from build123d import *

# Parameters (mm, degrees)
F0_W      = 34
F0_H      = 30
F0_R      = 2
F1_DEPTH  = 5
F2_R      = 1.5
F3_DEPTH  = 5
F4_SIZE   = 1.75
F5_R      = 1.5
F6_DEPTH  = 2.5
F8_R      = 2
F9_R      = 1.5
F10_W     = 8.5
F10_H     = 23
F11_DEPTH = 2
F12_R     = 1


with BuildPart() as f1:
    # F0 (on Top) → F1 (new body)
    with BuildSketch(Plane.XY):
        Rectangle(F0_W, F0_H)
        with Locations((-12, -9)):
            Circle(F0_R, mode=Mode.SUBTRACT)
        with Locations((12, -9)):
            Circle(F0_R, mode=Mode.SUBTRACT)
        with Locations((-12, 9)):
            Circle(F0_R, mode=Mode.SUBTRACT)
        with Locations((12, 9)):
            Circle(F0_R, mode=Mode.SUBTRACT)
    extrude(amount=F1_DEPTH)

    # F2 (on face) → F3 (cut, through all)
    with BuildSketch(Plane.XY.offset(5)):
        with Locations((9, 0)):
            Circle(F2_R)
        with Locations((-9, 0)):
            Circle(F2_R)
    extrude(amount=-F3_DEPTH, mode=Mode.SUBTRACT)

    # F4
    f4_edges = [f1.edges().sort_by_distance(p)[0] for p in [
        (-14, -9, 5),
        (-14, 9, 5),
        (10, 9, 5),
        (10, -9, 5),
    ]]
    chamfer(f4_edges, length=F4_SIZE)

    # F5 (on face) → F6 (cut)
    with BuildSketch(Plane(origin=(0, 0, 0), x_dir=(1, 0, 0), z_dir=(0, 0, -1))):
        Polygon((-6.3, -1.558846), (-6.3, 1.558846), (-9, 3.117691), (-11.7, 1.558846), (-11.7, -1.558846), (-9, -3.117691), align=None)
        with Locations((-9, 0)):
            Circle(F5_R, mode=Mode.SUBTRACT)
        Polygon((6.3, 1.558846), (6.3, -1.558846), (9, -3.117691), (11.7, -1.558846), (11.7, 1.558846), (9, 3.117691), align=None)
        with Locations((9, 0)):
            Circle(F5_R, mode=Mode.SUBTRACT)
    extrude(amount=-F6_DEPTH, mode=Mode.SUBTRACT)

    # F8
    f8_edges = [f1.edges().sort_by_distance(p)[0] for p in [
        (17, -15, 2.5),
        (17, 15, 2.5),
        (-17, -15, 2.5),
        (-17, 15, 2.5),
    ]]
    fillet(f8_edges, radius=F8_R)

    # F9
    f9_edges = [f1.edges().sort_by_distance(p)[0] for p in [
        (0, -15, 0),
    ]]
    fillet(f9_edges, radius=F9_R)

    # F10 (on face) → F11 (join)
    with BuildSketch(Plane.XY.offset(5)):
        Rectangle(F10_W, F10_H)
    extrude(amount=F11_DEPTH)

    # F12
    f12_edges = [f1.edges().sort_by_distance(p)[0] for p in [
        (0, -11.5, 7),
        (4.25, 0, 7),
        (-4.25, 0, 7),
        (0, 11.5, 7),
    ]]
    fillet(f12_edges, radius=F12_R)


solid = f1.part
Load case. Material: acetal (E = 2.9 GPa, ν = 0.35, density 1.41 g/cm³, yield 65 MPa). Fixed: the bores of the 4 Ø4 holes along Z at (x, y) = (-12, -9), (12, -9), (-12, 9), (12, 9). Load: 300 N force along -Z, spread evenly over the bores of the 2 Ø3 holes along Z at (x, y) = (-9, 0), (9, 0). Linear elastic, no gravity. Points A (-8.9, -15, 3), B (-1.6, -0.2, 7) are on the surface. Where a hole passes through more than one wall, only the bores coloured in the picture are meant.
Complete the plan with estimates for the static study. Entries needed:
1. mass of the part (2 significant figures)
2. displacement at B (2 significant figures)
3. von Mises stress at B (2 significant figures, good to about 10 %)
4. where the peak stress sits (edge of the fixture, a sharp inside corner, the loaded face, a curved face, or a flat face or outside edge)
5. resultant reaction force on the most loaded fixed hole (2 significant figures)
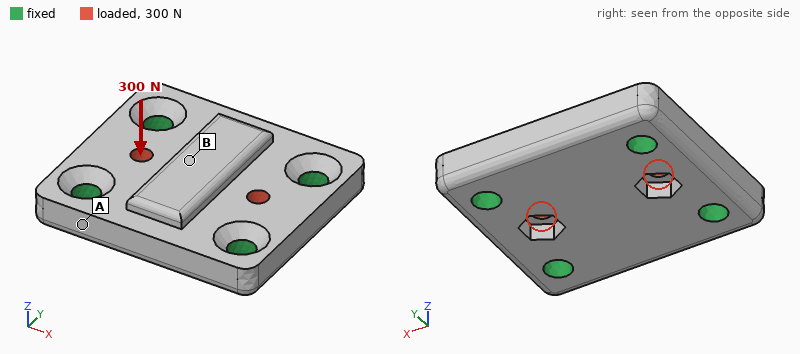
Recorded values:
6.9 g
23 µm
3.7 MPa
the loaded face
87 N
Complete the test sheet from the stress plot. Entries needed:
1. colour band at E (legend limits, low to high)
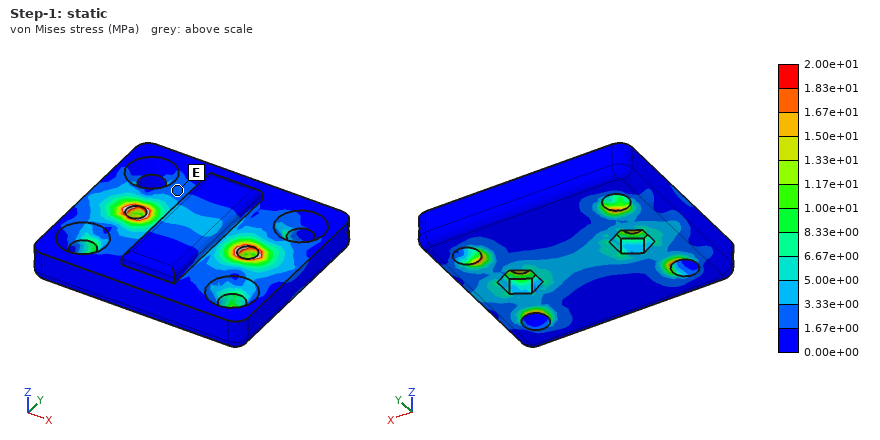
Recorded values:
1.67e+00 to 3.33e+00 MPa
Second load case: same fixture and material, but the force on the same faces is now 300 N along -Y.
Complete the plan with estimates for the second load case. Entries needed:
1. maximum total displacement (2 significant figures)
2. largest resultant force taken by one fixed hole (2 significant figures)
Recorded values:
12 µm
79 N
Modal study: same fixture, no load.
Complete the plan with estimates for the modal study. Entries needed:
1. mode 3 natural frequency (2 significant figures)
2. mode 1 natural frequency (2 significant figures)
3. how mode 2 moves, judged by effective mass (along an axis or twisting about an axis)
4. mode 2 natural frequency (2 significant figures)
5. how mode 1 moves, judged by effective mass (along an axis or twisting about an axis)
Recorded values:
14 kHz
8800 Hz
twisting about X
10 kHz
along Z
